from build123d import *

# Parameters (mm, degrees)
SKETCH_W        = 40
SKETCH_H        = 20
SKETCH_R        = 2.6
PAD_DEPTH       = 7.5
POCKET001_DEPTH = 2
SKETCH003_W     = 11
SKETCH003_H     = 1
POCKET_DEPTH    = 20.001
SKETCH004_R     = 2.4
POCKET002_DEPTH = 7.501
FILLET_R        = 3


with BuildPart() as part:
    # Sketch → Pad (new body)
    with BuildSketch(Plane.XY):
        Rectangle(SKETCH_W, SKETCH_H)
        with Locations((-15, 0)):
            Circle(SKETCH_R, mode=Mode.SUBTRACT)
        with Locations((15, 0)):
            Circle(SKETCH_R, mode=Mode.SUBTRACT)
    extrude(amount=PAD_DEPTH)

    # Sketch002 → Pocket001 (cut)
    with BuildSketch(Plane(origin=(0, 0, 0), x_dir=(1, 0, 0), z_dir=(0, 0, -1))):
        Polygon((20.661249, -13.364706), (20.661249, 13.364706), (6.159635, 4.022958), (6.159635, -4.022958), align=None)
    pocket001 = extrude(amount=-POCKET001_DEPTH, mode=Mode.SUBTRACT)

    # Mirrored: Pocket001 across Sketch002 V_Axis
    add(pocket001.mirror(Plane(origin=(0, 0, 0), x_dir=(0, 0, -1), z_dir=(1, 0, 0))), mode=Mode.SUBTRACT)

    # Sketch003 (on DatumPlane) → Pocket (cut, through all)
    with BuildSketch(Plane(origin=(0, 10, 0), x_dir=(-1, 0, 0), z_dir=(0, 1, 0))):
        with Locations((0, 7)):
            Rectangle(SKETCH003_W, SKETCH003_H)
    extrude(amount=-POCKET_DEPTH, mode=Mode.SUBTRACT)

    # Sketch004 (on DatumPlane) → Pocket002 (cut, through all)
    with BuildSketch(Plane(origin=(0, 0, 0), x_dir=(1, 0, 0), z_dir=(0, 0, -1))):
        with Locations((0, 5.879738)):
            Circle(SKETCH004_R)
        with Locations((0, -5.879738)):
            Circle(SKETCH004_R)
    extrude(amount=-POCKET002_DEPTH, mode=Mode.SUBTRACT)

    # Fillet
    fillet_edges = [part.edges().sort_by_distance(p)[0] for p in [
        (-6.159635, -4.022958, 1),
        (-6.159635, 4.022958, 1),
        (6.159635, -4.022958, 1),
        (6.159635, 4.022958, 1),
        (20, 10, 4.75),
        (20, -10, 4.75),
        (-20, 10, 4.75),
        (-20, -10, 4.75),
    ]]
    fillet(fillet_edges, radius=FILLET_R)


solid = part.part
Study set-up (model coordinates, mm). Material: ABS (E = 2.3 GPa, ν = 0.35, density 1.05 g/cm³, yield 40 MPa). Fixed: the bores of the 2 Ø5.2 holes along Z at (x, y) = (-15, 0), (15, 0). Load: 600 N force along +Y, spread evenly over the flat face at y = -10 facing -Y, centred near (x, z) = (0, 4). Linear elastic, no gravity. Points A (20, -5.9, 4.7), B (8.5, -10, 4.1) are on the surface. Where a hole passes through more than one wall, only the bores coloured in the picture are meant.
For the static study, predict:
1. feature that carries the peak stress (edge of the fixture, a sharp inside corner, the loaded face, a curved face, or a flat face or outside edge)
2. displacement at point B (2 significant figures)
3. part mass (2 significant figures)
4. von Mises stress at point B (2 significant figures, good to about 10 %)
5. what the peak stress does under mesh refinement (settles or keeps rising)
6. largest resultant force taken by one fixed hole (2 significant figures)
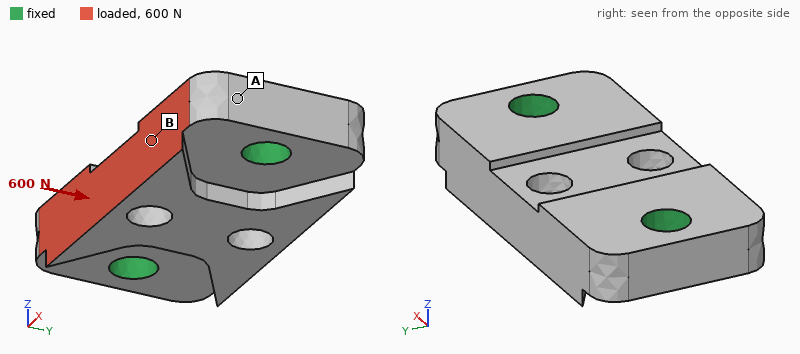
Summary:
edge of the fixture
46 µm
4.6 g
4.0 MPa
keeps rising
300 N
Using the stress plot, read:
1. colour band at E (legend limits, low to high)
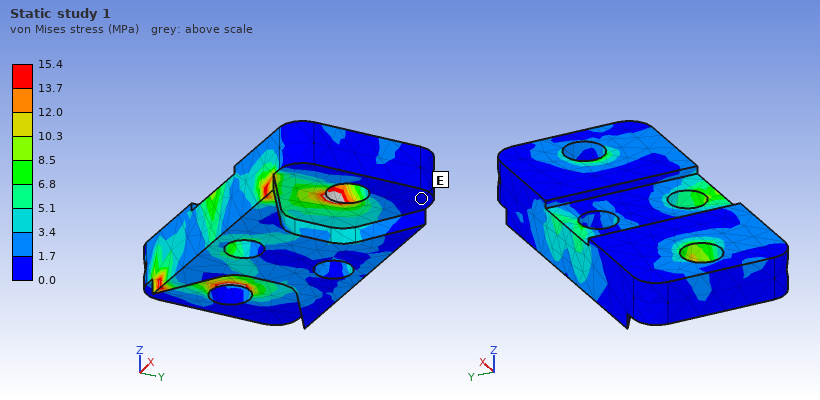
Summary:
0.0 to 1.7 MPa
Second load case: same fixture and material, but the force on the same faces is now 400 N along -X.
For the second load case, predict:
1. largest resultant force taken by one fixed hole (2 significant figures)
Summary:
230 N
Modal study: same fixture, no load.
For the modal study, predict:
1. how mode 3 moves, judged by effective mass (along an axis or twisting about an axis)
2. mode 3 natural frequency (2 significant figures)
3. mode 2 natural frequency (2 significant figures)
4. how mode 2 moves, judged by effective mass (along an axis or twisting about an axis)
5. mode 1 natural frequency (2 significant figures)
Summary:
along Y
11 kHz
7800 Hz
along Z
7300 Hz
